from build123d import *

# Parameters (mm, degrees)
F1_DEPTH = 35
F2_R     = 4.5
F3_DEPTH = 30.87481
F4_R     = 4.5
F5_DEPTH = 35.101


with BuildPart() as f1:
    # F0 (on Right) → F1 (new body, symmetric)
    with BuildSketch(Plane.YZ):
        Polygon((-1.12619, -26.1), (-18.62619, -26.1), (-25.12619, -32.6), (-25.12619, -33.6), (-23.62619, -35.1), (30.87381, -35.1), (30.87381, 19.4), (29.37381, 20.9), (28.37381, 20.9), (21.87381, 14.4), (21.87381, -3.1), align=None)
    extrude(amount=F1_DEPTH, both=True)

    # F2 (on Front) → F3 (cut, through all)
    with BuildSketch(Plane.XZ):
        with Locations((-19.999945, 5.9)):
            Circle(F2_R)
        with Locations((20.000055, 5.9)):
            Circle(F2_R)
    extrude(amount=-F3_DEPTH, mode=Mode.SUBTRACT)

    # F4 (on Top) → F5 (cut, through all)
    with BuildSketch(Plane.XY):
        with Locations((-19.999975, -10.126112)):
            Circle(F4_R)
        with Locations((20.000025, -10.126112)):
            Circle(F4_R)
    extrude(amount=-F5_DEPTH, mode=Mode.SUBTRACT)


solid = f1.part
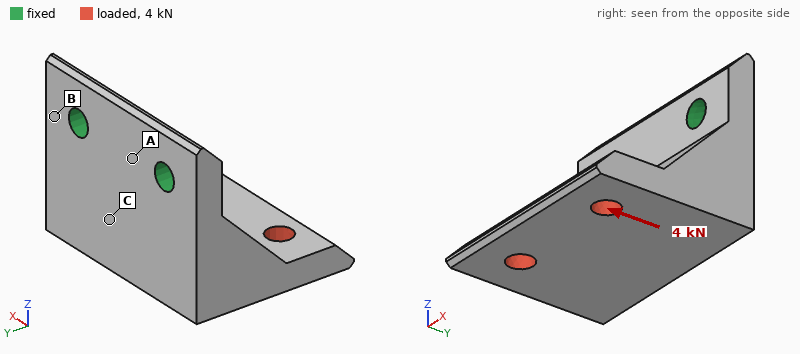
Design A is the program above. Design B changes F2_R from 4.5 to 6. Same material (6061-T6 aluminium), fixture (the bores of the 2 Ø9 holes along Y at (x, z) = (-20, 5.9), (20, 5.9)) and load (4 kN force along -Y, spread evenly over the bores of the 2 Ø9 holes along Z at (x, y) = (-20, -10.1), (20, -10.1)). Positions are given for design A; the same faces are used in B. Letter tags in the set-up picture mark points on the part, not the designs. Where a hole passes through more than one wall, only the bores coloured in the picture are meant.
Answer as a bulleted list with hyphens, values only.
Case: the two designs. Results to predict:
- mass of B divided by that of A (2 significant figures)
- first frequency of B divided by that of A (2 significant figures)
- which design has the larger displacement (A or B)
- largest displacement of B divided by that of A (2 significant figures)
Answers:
- 0.99
- 1.1
- A
- 0.82
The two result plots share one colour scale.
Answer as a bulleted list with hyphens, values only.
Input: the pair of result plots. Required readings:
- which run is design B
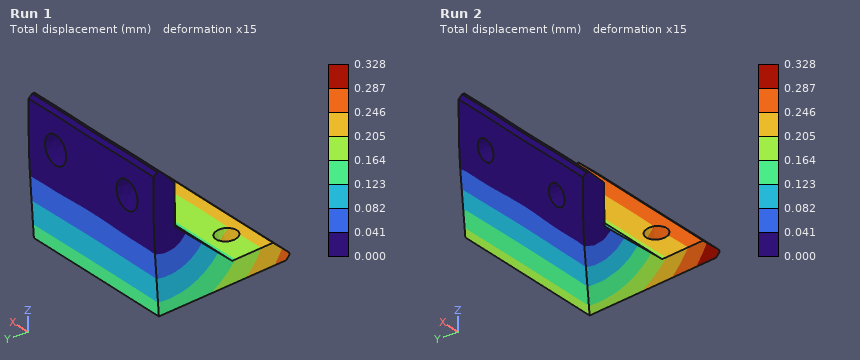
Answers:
- Run 1
